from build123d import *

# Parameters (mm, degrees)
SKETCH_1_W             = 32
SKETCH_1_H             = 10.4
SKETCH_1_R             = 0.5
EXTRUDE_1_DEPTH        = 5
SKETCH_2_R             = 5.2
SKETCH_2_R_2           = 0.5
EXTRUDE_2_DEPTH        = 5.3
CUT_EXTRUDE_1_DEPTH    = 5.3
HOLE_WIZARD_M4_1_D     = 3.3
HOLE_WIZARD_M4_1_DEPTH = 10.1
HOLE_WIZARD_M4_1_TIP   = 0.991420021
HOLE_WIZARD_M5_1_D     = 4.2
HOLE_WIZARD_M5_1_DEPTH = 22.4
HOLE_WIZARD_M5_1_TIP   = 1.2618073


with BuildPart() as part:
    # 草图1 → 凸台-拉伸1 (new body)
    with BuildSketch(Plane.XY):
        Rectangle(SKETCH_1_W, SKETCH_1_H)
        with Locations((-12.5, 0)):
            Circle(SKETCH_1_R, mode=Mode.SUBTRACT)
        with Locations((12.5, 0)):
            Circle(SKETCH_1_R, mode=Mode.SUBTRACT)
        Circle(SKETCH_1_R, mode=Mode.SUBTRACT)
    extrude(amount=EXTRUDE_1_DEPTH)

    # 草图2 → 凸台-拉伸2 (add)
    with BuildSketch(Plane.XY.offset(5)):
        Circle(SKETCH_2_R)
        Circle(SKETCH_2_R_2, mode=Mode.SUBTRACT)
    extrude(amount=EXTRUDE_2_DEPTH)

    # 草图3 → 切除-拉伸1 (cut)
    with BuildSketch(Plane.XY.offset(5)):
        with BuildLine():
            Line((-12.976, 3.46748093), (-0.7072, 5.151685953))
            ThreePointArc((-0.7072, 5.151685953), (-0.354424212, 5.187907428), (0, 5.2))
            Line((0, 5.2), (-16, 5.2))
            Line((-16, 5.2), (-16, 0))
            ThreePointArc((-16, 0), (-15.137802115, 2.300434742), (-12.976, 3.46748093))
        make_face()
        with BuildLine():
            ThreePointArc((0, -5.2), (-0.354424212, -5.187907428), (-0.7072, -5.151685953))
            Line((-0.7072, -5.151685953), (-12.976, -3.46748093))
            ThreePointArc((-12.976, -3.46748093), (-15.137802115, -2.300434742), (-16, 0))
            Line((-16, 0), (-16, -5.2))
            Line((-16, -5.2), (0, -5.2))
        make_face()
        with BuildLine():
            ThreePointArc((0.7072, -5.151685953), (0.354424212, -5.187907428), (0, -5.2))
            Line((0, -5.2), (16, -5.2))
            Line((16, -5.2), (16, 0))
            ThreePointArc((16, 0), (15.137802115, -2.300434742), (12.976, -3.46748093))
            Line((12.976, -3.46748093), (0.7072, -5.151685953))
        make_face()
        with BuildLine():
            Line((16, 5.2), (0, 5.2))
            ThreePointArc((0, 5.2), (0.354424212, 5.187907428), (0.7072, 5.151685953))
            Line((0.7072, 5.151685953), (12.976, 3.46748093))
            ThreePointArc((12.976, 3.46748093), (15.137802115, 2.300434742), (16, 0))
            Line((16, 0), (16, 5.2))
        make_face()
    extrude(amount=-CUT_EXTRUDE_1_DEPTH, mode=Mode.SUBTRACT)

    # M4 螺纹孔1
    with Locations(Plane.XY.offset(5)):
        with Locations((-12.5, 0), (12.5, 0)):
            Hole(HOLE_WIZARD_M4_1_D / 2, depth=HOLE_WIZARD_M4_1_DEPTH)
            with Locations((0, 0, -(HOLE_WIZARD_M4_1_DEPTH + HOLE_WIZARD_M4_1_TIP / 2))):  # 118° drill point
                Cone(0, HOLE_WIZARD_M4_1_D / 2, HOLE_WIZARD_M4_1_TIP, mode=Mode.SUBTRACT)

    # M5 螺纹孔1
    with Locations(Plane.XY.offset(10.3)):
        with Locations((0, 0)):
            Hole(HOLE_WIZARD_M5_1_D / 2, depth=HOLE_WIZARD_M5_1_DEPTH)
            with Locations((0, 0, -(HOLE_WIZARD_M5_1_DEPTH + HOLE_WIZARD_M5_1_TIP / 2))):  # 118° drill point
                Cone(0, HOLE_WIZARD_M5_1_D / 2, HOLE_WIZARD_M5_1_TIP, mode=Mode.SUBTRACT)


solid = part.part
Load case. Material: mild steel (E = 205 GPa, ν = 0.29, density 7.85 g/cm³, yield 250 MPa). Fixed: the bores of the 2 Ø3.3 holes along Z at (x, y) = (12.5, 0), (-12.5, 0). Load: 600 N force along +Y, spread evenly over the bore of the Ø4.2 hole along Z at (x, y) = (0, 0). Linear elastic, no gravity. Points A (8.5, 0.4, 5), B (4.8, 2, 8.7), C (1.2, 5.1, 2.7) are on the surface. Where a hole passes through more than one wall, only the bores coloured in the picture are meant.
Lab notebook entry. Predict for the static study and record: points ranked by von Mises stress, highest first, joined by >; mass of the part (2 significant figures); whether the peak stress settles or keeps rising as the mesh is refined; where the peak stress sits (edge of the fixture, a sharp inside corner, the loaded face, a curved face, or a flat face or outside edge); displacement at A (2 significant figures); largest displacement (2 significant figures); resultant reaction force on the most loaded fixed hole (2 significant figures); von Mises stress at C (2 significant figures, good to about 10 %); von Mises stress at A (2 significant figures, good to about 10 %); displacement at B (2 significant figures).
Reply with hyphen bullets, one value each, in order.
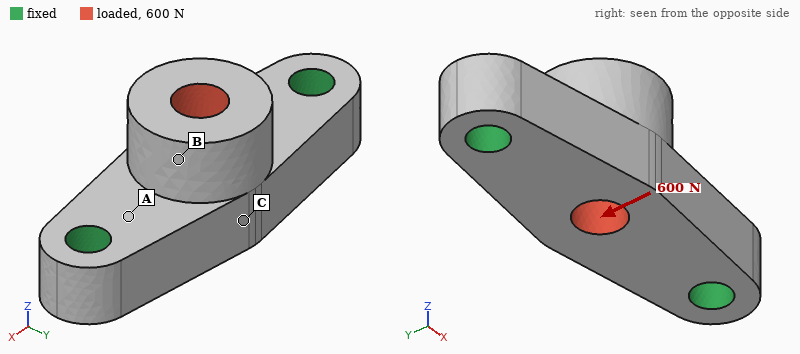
- A > C > B
- 12 g
- keeps rising
- edge of the fixture
- 1.0 µm
- 5.3 µm
- 300 N
- 21 MPa
- 43 MPa
- 4.2 µm
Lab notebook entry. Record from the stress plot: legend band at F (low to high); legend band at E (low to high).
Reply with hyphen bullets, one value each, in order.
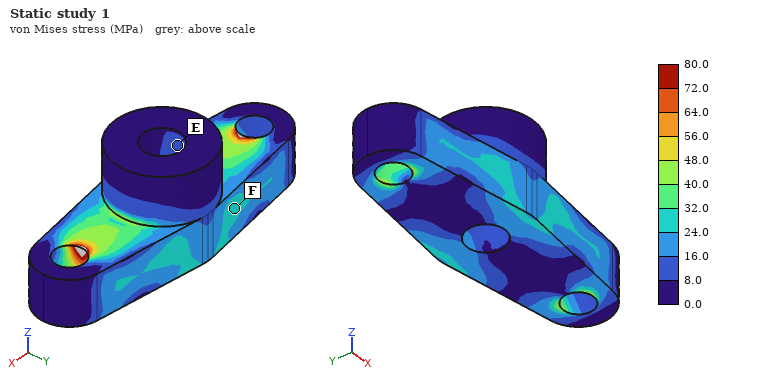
- 24.0 to 32.0 MPa
- 8.0 to 16.0 MPa
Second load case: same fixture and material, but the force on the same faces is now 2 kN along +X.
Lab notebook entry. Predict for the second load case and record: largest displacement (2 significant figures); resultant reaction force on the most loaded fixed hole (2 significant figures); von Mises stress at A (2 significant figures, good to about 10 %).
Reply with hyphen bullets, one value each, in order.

- 3.8 µm
- 1.0 kN
- 37 MPa
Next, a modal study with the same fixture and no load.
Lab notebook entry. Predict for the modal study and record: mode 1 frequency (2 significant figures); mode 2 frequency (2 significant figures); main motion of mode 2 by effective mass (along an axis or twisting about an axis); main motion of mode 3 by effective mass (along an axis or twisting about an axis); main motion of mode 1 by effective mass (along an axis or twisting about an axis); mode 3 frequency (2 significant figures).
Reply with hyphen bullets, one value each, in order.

- 24 kHz
- 32 kHz
- along Z
- along Y
- along Y
- 44 kHz
